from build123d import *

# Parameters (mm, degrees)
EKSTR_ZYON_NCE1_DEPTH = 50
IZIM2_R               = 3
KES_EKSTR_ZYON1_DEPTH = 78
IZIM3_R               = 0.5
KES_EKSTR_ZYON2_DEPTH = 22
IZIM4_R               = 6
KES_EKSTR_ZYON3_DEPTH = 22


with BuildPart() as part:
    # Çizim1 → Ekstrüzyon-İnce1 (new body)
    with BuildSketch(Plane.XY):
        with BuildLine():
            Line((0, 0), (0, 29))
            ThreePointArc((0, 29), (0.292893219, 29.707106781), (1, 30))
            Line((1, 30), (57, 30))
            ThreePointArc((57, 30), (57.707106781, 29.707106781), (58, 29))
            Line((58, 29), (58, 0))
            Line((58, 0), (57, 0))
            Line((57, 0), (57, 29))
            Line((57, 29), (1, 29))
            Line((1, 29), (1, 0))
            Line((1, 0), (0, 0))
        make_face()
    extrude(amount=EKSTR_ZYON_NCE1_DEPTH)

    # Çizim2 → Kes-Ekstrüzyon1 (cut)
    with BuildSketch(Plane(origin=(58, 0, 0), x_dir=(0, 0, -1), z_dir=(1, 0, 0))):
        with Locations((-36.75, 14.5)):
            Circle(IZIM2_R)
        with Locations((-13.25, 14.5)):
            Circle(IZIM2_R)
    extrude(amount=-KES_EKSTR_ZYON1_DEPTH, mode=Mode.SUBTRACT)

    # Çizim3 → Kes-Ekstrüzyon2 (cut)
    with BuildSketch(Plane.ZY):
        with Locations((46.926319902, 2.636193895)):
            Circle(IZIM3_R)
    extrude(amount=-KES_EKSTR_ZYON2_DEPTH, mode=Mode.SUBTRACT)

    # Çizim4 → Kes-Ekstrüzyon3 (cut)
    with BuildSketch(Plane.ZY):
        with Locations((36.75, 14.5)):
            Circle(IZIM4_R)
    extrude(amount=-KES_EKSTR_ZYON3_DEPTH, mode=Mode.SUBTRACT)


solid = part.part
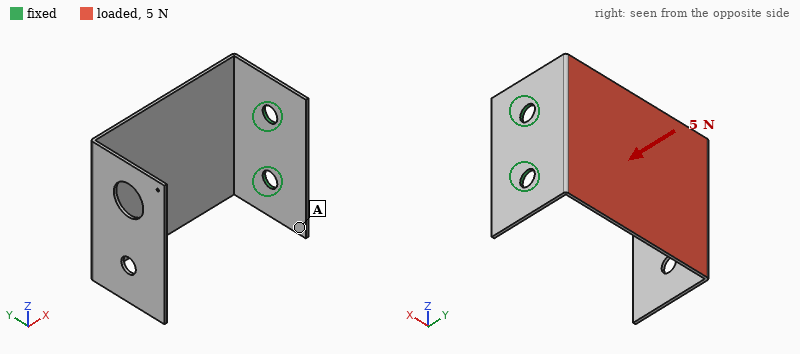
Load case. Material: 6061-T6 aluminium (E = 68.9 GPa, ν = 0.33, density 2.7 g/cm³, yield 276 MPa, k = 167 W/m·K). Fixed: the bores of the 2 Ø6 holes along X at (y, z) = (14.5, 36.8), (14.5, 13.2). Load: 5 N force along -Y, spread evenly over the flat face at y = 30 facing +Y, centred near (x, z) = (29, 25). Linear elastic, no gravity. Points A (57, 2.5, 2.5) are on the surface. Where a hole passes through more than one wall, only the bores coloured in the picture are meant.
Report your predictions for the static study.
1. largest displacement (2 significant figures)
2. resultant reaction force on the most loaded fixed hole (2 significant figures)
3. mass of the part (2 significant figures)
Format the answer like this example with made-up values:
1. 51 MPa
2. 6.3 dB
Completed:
1. 0.82 mm
2. 2.6 N
3. 15 g
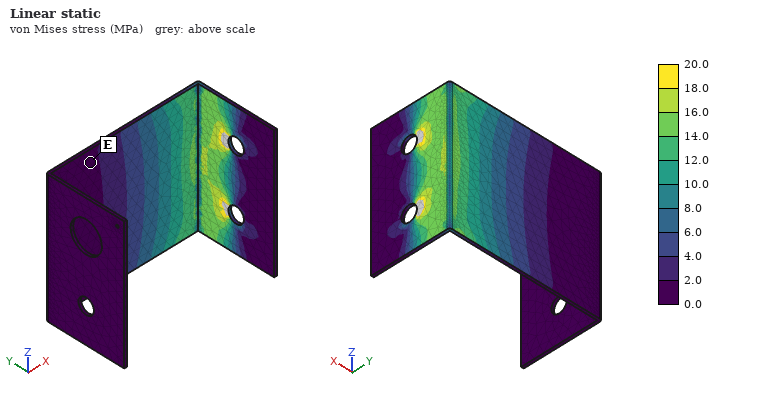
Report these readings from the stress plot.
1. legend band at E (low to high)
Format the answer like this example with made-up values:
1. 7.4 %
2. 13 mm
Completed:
1. 0.0 to 2.0 MPa
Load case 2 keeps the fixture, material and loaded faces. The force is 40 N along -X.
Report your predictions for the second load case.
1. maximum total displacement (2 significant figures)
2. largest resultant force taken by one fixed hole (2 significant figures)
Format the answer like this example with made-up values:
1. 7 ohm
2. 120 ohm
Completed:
1. 0.86 mm
2. 20 N
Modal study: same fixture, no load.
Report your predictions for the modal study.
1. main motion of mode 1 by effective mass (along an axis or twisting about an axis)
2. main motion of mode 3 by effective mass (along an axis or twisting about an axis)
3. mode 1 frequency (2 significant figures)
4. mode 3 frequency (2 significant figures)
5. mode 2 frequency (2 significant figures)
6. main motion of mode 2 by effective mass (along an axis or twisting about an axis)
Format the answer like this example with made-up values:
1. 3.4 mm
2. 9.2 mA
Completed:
1. along Y
2. along X
3. 110 Hz
4. 460 Hz
5. 260 Hz
6. along Z
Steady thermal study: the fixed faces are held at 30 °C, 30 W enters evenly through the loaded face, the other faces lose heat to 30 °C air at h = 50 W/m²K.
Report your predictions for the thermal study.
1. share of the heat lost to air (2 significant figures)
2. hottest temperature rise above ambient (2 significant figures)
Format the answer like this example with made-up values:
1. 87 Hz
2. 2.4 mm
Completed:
1. 53 %
2. 62 K
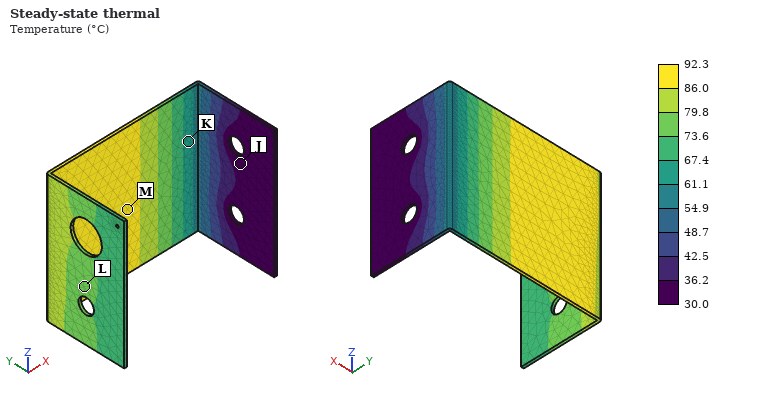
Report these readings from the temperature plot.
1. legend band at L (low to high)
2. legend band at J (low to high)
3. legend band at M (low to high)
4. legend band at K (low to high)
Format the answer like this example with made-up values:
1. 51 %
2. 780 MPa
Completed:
1. 73.6 to 79.8 °C
2. 30.0 to 36.2 °C
3. 86.0 to 92.3 °C
4. 61.1 to 67.4 °C
